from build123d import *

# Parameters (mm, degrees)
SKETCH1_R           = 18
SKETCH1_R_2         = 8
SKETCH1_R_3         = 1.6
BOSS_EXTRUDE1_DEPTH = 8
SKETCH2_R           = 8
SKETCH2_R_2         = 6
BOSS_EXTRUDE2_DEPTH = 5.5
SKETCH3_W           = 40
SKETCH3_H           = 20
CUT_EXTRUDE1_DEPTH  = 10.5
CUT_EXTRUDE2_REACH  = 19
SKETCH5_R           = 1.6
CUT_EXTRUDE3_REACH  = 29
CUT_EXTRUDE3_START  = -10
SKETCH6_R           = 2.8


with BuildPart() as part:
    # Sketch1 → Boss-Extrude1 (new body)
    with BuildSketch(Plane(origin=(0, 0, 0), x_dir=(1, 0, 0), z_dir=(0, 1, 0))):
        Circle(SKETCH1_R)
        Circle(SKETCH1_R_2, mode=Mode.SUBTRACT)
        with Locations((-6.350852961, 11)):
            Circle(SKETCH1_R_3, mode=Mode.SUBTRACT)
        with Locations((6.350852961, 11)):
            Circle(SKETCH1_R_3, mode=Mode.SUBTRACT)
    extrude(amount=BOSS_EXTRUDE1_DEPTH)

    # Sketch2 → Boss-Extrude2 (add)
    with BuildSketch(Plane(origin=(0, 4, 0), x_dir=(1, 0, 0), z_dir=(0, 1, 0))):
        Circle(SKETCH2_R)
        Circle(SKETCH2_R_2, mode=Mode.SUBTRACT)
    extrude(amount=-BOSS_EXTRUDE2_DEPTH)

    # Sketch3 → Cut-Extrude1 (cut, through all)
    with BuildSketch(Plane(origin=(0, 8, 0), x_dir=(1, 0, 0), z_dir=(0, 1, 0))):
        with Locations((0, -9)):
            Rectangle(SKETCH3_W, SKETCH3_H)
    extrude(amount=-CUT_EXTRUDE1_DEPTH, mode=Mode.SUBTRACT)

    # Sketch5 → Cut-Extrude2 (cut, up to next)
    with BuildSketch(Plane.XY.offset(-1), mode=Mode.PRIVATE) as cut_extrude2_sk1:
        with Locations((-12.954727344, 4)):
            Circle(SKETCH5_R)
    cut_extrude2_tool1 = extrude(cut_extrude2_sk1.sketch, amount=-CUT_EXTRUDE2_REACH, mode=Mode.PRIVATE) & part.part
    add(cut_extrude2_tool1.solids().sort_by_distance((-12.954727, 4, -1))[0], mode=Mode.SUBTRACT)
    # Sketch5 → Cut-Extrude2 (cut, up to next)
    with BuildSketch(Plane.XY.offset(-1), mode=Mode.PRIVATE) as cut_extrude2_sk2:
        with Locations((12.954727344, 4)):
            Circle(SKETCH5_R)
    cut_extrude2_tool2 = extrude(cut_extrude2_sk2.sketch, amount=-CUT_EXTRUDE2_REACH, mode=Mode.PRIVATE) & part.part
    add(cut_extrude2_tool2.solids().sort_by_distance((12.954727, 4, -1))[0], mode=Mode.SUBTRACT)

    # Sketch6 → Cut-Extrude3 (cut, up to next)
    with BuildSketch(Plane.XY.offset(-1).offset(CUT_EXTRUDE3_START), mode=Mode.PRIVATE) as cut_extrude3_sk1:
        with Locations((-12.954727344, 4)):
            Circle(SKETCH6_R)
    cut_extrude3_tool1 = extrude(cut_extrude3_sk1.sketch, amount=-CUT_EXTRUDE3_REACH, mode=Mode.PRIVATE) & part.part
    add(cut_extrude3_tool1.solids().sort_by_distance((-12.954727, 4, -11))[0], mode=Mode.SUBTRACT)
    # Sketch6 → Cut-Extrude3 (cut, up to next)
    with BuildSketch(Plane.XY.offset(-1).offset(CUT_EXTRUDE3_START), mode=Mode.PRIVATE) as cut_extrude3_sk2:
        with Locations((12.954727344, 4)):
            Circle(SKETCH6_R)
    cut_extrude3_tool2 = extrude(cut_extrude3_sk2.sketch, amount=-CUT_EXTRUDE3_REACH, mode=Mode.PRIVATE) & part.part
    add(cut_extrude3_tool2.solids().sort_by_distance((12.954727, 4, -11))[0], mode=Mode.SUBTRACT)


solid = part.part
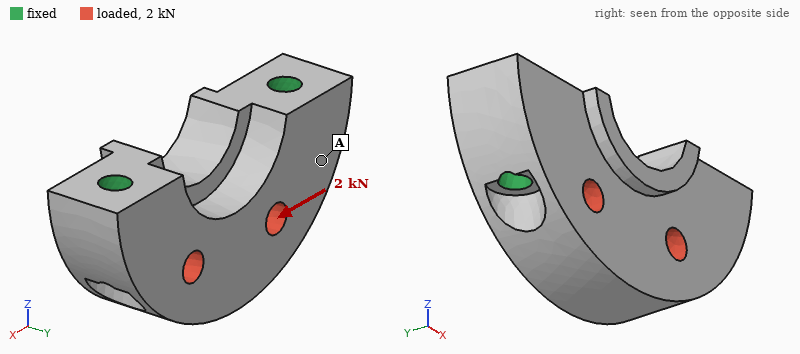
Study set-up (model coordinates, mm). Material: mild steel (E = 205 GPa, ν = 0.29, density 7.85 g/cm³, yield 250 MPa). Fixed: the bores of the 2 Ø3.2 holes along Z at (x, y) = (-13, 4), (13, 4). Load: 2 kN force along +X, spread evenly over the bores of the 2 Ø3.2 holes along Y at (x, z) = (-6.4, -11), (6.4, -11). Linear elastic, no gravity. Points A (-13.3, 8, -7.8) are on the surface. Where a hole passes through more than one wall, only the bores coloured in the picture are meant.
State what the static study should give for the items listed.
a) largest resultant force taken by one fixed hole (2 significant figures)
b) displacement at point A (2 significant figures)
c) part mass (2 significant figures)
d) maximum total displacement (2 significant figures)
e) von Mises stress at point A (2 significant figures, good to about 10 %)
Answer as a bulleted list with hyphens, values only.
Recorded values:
- 1.0 kN
- 0.16 µm
- 23 g
- 1.0 µm
- 6.9 MPa
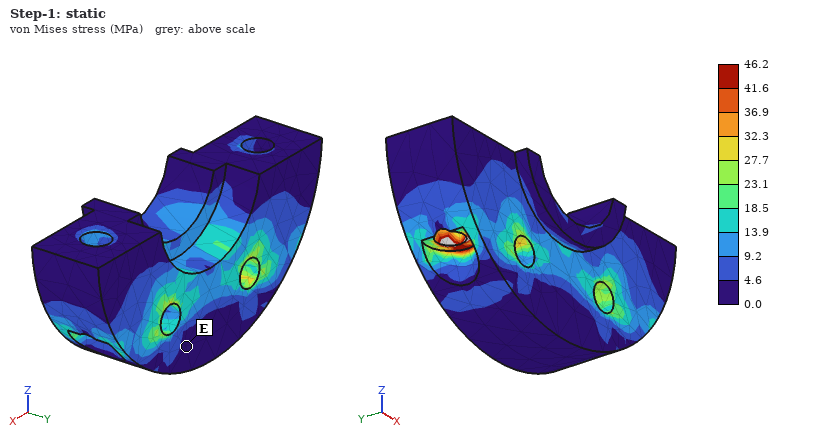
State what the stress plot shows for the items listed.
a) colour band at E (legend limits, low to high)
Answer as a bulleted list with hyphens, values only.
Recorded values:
- 0.0 to 4.6 MPa
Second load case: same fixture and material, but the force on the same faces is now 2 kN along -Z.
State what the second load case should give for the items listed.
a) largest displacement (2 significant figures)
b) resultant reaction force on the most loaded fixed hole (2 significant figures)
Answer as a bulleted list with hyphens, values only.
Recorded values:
- 1.5 µm
- 1.1 kN
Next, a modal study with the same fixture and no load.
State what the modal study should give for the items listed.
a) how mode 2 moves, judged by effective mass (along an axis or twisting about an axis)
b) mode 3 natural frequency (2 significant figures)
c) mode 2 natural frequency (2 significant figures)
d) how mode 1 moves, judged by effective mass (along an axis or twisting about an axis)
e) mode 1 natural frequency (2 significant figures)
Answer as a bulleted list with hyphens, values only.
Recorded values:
- along Z
- 55 kHz
- 49 kHz
- along Y
- 27 kHz
